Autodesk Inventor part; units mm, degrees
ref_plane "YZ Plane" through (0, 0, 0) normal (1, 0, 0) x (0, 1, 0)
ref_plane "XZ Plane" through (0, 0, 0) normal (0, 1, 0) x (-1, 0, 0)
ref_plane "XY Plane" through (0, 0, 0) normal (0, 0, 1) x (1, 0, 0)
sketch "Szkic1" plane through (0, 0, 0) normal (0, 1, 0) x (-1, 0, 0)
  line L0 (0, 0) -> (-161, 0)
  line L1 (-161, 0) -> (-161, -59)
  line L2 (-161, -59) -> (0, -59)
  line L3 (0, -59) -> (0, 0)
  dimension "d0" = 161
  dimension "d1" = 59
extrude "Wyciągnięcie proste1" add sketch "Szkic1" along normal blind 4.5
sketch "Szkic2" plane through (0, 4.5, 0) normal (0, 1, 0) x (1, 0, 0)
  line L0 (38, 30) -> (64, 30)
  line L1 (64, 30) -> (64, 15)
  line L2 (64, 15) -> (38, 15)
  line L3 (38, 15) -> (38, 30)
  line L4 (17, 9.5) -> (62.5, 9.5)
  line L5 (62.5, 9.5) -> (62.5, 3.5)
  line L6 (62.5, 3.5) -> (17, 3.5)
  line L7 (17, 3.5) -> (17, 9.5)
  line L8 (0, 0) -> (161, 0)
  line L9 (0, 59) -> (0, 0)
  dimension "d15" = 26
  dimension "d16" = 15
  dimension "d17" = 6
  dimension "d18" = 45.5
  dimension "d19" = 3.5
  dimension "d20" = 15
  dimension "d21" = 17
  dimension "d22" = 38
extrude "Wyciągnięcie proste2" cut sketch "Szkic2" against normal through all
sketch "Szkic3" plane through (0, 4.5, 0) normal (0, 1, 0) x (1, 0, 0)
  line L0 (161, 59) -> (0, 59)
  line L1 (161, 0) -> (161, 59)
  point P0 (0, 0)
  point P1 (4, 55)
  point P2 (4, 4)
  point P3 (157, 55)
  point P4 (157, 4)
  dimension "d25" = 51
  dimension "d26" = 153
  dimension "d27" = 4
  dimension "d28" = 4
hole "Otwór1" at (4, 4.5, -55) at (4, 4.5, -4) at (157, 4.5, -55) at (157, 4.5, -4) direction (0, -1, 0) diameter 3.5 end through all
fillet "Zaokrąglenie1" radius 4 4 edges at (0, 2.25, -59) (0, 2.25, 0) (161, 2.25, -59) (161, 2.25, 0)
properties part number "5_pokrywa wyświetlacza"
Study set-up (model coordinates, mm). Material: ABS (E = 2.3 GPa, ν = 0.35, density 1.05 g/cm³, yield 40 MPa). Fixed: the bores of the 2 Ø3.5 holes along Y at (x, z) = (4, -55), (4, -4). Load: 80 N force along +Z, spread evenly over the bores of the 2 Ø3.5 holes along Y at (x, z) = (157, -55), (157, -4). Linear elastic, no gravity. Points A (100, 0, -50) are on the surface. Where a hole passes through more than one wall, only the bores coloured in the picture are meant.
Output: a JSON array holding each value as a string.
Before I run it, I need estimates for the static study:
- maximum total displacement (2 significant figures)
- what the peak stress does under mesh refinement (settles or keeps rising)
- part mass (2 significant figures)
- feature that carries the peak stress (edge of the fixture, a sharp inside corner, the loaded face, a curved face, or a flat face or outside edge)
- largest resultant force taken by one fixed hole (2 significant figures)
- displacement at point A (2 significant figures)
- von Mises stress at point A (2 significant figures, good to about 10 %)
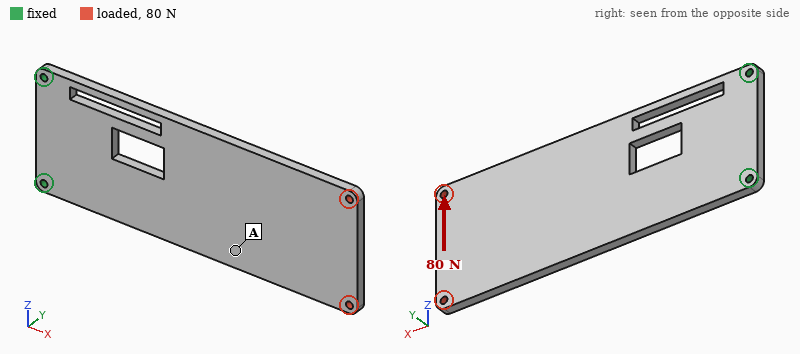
["0.88 mm", "keeps rising", "42 g", "edge of the fixture", "250 N", "0.44 mm", "1.2 MPa"]
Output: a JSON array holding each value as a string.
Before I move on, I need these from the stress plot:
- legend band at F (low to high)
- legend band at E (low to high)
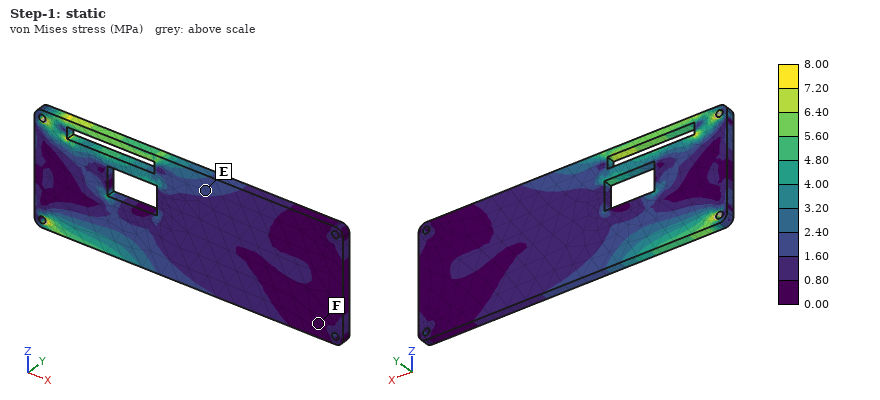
["0.00 to 0.80 MPa", "1.60 to 2.40 MPa"]
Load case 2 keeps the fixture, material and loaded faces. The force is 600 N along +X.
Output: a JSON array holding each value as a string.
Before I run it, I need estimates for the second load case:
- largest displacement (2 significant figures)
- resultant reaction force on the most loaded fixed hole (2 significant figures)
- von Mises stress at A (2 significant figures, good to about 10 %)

["0.39 mm", "320 N", "2.3 MPa"]
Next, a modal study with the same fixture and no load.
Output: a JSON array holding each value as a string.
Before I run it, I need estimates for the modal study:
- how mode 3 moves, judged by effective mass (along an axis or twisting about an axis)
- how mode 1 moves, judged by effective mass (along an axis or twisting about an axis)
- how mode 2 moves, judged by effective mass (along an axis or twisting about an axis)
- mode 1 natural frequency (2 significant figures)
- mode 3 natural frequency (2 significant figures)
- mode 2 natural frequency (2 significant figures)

["along Y", "along Y", "twisting about X", "36 Hz", "250 Hz", "210 Hz"]
